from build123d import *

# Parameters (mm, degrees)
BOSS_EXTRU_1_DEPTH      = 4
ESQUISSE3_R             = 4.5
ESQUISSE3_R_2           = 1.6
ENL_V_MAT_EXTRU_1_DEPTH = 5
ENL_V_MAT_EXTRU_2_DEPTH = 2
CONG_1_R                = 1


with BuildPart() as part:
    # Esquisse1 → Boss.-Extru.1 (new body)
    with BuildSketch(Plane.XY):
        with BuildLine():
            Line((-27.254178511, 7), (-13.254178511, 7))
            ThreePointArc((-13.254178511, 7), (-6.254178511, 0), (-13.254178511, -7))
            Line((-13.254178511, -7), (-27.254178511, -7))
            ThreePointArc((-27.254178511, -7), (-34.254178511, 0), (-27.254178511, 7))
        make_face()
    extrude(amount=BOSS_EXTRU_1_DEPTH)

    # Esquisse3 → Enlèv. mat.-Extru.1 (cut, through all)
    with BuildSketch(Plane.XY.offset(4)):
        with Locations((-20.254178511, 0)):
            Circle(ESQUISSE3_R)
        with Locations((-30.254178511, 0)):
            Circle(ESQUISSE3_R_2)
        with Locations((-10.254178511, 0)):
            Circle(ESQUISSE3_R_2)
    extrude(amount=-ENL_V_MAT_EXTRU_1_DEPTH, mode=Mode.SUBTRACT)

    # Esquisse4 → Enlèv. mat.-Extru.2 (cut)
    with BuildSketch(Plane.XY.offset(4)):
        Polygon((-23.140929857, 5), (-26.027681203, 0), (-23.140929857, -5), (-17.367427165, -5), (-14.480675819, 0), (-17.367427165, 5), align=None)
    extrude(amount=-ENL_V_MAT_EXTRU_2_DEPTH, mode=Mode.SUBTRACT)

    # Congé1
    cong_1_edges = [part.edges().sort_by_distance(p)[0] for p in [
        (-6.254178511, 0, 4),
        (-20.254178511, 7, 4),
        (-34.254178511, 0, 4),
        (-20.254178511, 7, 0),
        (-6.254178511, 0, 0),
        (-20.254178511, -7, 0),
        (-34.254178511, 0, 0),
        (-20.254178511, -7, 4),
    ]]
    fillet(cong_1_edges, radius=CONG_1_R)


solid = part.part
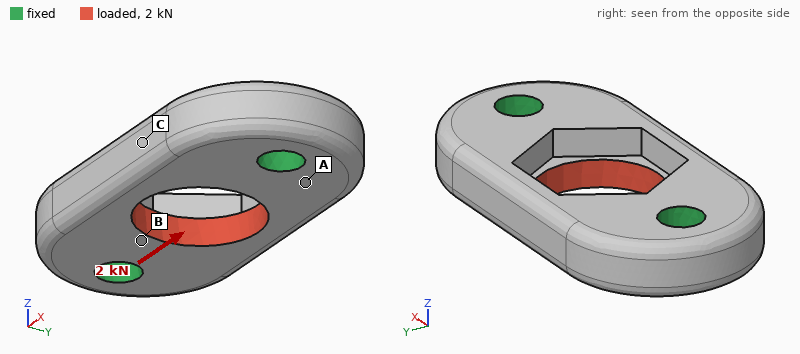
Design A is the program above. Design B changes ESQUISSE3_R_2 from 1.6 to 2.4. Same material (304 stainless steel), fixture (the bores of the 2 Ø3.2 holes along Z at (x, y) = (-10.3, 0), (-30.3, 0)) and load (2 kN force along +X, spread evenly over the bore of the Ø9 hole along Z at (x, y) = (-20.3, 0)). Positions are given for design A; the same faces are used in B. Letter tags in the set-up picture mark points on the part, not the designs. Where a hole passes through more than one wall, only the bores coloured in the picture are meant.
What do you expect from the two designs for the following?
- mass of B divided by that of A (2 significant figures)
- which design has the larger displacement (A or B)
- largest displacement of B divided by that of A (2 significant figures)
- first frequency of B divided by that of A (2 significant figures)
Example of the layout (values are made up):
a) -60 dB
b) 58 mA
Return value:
a) 0.92
b) A
c) 0.88
d) 1.2
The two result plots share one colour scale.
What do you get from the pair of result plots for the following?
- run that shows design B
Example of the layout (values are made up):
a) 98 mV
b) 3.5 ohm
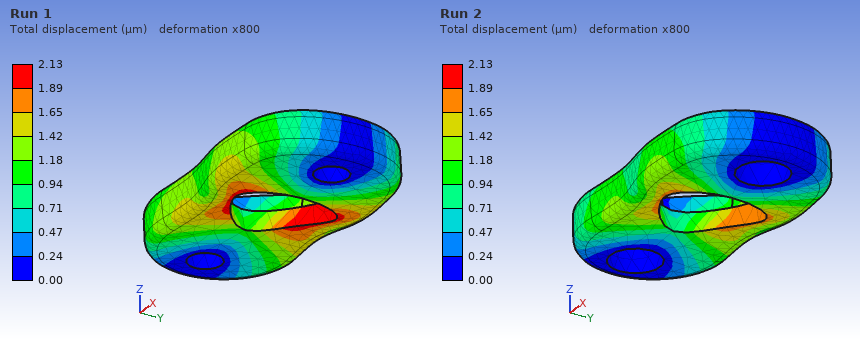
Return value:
a) Run 2
